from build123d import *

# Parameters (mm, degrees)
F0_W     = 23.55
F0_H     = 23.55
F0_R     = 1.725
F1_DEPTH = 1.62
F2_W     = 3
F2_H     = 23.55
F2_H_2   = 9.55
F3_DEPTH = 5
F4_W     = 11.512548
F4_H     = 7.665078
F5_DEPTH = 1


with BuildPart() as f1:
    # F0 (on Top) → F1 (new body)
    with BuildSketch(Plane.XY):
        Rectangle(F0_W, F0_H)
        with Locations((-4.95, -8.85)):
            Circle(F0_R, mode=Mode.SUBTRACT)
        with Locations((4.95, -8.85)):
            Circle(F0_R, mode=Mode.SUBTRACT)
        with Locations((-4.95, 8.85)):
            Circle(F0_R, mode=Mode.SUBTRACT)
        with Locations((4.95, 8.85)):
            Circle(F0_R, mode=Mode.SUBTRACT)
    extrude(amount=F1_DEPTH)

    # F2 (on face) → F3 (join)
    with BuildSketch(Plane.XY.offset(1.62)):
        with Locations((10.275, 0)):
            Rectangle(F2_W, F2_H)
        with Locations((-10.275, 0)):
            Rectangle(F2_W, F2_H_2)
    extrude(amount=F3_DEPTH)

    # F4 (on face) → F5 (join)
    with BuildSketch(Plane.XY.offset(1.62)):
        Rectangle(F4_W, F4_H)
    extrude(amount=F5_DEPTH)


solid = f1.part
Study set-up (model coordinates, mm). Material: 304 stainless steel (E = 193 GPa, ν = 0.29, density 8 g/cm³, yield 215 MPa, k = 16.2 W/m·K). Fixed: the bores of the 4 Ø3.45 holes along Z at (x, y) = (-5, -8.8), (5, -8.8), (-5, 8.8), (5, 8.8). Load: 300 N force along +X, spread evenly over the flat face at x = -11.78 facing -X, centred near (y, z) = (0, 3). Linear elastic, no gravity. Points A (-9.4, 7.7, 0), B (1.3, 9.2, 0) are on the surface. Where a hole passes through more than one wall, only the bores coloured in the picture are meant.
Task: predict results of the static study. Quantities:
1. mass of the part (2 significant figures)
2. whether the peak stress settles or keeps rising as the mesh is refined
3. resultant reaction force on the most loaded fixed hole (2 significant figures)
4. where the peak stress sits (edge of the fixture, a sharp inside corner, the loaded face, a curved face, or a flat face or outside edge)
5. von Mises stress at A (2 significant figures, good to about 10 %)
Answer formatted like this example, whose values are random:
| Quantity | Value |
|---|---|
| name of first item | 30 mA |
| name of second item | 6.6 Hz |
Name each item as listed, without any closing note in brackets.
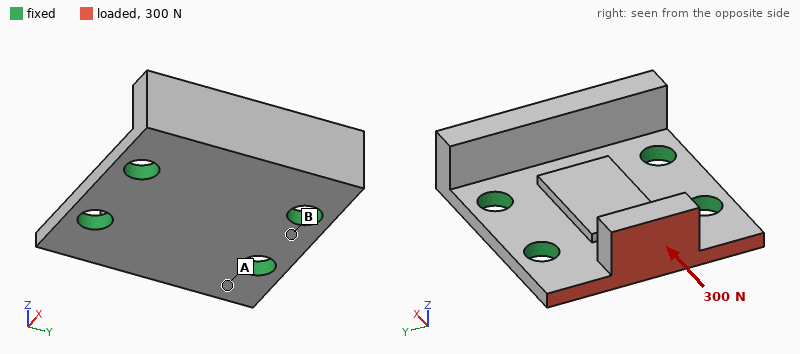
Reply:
| Quantity | Value |
|---|---|
| mass of the part | 11 g |
| whether the peak stress settles or keeps rising as the mesh is refined | keeps rising |
| resultant reaction force on the most loaded fixed hole | 100 N |
| where the peak stress sits | edge of the fixture |
| von Mises stress at A | 34 MPa |
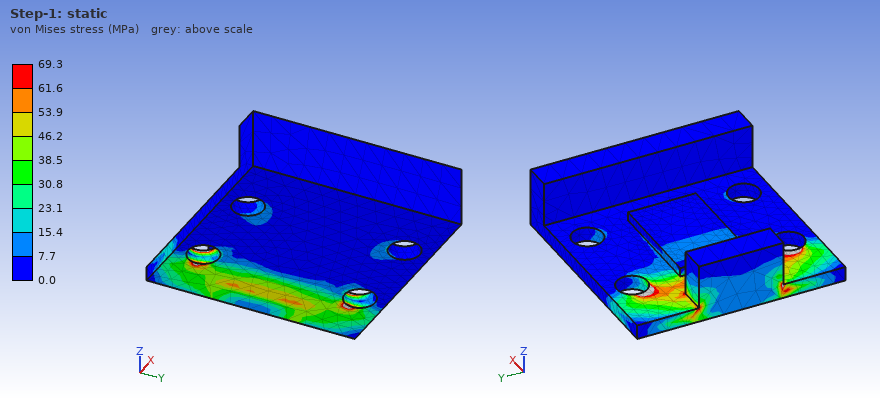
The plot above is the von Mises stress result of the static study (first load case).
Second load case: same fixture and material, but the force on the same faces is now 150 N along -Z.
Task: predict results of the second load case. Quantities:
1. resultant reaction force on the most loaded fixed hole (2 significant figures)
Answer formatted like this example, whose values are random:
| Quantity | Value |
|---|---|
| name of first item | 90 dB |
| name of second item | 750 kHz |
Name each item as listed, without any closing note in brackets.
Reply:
| Quantity | Value |
|---|---|
| resultant reaction force on the most loaded fixed hole | 92 N |
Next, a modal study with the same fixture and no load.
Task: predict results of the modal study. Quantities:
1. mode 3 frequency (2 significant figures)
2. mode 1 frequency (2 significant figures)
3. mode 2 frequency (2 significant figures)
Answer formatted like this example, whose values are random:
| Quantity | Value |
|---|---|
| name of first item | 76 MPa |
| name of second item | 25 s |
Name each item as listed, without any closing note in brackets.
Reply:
| Quantity | Value |
|---|---|
| mode 3 frequency | 25 kHz |
| mode 1 frequency | 13 kHz |
| mode 2 frequency | 15 kHz |
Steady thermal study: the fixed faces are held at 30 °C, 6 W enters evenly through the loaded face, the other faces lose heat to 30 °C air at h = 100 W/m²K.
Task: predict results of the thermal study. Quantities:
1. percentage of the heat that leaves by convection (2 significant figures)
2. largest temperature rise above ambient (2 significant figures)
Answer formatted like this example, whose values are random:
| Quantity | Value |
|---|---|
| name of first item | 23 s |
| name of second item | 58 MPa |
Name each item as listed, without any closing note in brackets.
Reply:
| Quantity | Value |
|---|---|
| percentage of the heat that leaves by convection | 30 % |
| largest temperature rise above ambient | 76 K |
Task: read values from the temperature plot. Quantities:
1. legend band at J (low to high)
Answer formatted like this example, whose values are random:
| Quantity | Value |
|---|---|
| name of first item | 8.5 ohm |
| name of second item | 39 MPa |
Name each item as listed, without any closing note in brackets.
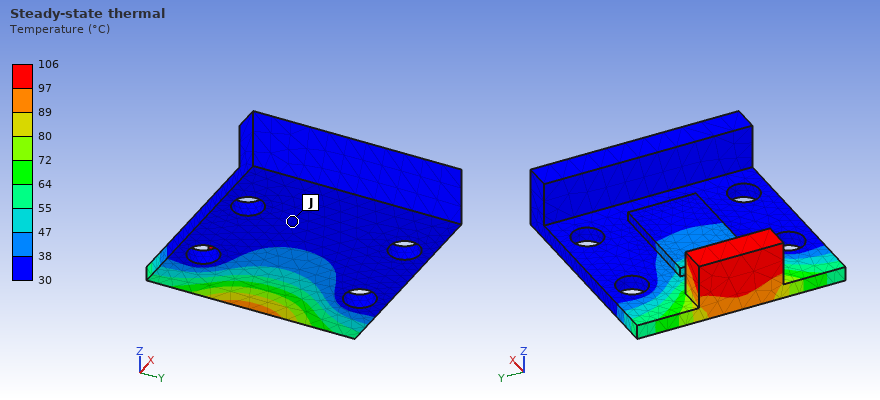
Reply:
| Quantity | Value |
|---|---|
| legend band at J | 30 to 38 °C |
